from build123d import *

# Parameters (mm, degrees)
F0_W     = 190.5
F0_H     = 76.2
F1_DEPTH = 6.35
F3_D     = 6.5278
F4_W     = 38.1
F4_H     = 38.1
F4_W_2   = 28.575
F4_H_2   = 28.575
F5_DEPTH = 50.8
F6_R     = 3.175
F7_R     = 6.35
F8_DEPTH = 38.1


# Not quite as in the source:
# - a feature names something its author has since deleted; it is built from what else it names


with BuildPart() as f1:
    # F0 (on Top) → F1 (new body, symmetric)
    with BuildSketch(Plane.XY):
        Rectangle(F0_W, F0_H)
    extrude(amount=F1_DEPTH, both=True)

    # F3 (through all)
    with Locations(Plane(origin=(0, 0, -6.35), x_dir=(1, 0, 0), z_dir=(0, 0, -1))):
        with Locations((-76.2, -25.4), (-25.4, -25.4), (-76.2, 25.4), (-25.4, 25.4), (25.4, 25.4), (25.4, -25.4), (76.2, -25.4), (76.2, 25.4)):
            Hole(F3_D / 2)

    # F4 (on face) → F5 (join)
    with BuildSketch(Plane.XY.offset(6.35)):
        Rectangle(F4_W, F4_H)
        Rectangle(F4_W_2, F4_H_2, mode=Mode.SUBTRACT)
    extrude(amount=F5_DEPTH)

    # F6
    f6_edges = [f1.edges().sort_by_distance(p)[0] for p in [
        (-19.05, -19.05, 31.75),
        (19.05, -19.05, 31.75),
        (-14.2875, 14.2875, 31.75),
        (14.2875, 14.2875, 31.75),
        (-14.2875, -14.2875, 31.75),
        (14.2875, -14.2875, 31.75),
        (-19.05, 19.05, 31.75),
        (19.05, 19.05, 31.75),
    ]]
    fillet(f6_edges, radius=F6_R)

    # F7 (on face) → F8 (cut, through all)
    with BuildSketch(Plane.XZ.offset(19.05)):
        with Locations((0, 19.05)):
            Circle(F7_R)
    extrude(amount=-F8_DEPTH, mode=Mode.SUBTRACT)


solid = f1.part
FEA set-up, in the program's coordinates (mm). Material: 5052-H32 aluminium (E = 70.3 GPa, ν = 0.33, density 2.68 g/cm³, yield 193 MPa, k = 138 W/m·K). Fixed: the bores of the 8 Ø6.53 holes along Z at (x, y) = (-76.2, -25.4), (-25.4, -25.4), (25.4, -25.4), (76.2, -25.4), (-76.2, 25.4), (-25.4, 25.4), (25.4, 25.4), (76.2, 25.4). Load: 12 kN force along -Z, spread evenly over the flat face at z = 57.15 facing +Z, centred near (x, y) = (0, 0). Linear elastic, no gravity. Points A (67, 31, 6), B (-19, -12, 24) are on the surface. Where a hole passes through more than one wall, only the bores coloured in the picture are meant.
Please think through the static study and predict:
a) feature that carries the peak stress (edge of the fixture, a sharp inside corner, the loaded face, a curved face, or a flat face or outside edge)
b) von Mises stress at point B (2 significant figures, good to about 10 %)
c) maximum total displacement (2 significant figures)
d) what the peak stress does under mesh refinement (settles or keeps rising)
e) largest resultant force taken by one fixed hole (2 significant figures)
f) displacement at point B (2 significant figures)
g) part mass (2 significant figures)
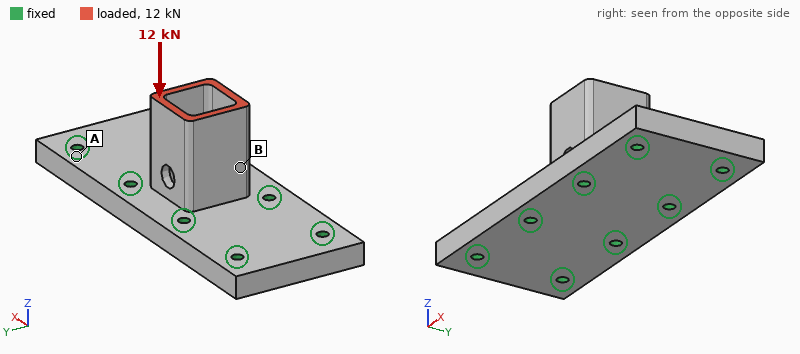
edge of the fixture
19 MPa
26 µm
keeps rising
3.1 kN
16 µm
570 g
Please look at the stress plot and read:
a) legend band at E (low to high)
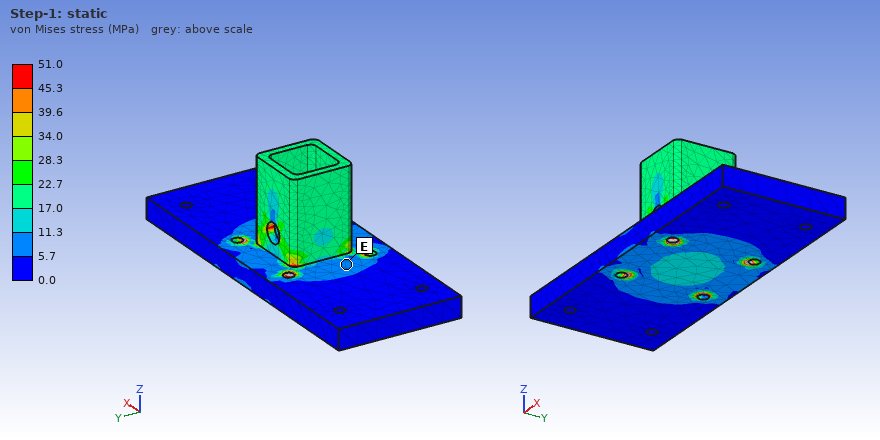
5.7 to 11.3 MPa
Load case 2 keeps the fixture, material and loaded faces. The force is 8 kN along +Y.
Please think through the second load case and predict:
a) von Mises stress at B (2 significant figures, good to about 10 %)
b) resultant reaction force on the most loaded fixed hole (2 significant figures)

44 MPa
5.4 kN
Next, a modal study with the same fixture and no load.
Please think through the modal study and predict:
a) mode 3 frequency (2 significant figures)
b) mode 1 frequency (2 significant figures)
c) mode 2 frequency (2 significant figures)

9100 Hz
6200 Hz
6500 Hz
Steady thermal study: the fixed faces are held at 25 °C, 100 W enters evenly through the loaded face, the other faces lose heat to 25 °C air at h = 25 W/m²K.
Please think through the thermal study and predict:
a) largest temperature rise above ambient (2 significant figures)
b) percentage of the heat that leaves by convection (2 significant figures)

66 K
13 %
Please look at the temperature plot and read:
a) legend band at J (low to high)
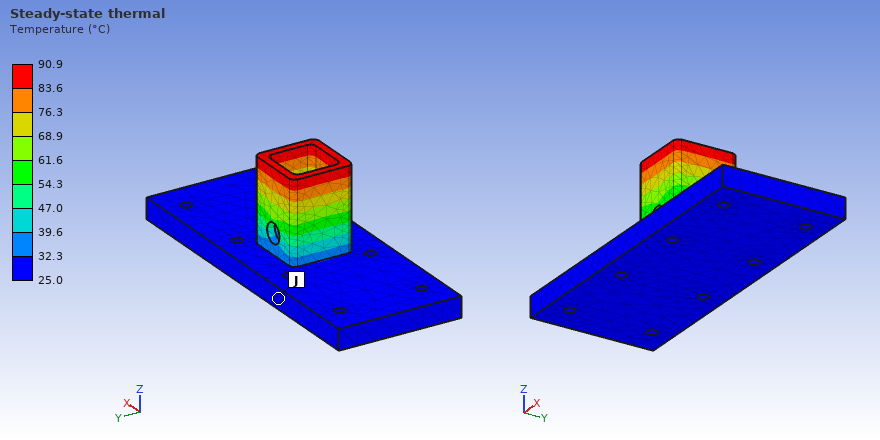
25.0 to 32.3 °C
